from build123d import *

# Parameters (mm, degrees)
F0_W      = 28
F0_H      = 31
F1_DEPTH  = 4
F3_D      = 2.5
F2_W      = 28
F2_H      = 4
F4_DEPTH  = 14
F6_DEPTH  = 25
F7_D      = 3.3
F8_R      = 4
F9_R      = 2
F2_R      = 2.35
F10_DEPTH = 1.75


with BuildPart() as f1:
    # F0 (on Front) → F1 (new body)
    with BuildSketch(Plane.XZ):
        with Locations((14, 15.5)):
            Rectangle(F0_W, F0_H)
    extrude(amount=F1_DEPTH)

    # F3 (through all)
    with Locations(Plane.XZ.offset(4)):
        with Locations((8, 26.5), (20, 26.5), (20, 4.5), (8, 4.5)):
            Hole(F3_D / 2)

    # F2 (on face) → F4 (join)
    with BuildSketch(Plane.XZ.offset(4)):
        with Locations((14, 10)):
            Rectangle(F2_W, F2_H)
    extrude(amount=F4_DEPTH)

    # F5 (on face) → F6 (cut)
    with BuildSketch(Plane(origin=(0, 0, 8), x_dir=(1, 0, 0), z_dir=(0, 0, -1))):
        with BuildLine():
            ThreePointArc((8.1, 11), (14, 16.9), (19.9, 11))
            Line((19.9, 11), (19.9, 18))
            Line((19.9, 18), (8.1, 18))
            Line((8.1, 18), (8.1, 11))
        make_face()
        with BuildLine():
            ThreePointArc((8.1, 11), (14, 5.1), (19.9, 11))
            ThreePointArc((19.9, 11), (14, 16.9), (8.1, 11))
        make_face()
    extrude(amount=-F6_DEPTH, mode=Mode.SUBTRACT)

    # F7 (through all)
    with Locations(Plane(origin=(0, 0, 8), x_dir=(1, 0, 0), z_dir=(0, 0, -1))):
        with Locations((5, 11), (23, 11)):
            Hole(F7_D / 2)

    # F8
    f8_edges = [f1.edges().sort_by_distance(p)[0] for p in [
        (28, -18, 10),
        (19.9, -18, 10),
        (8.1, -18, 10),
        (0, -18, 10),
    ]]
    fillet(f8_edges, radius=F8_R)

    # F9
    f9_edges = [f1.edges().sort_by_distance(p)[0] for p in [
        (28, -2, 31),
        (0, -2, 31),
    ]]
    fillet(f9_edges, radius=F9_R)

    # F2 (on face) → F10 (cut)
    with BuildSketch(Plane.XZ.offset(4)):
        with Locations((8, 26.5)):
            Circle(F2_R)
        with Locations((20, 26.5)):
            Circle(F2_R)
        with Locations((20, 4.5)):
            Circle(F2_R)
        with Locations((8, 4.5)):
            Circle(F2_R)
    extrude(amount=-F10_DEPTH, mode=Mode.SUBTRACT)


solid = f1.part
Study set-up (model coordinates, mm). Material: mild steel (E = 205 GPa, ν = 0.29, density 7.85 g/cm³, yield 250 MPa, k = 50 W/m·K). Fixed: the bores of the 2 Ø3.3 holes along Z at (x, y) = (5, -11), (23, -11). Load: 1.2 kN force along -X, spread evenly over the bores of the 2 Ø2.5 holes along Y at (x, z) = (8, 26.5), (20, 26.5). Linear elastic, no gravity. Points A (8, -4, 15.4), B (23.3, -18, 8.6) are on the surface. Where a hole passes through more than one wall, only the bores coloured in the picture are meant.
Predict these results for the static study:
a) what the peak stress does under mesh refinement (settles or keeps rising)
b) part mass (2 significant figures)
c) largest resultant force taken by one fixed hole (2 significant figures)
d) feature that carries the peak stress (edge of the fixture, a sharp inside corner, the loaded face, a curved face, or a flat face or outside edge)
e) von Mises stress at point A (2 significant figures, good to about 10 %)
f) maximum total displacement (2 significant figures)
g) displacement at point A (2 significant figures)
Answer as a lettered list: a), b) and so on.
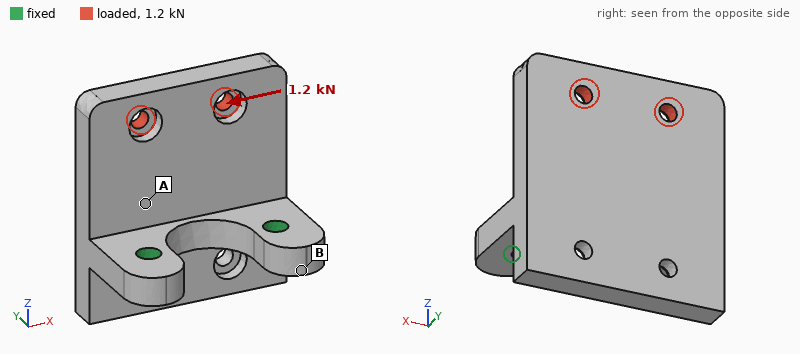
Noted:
a) keeps rising
b) 33 g
c) 1.2 kN
d) edge of the fixture
e) 53 MPa
f) 29 µm
g) 10 µm
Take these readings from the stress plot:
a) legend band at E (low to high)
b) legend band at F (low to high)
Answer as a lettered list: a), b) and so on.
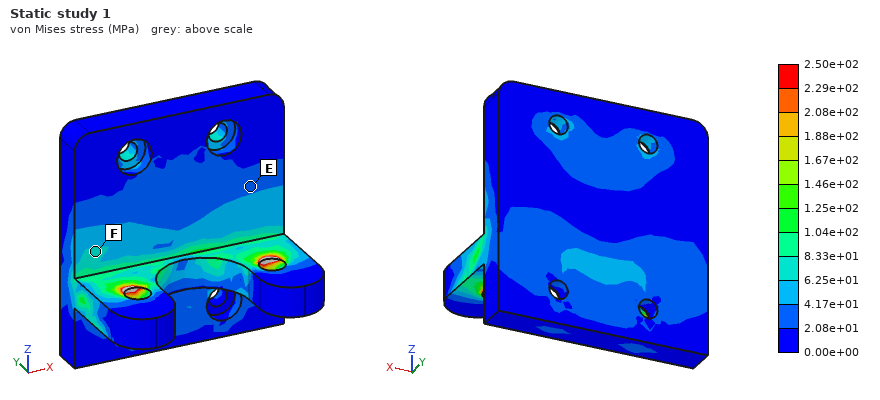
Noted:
a) 2.08e+01 to 4.17e+01 MPa
b) 6.25e+01 to 8.33e+01 MPa
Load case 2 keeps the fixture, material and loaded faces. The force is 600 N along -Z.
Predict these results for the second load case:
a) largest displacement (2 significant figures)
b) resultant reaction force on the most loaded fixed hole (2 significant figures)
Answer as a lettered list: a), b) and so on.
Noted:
a) 32 µm
b) 300 N
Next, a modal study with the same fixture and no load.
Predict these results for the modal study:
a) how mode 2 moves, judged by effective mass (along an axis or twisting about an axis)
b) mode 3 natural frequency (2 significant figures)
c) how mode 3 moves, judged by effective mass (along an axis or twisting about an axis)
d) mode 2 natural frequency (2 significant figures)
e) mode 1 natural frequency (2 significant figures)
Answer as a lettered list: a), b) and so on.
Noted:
a) along X
b) 14 kHz
c) along Z
d) 9500 Hz
e) 4100 Hz
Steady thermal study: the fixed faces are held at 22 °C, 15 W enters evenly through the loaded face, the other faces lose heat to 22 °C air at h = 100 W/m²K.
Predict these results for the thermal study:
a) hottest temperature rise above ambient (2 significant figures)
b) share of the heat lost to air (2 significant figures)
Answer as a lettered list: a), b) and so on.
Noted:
a) 60 K
b) 44 %
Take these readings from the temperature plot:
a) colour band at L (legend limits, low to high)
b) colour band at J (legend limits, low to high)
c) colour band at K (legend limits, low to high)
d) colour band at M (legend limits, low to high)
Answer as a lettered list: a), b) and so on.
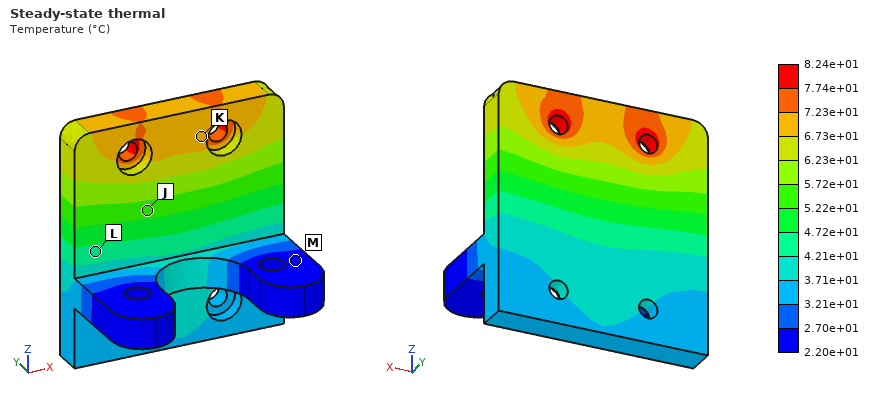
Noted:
a) 4.21e+01 to 4.72e+01 °C
b) 5.22e+01 to 5.72e+01 °C
c) 6.73e+01 to 7.23e+01 °C
d) 2.20e+01 to 2.70e+01 °C
